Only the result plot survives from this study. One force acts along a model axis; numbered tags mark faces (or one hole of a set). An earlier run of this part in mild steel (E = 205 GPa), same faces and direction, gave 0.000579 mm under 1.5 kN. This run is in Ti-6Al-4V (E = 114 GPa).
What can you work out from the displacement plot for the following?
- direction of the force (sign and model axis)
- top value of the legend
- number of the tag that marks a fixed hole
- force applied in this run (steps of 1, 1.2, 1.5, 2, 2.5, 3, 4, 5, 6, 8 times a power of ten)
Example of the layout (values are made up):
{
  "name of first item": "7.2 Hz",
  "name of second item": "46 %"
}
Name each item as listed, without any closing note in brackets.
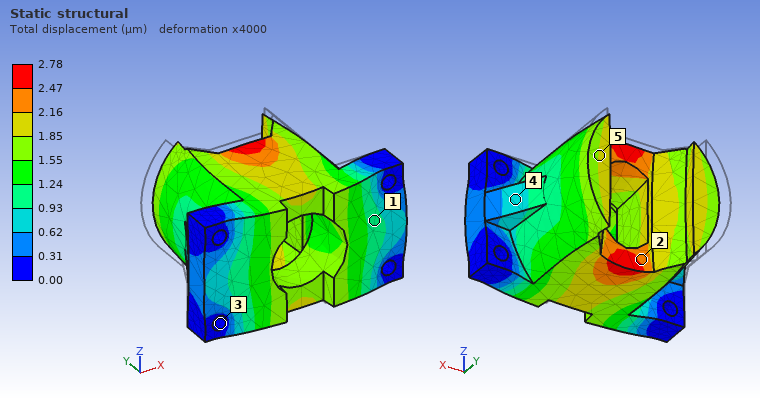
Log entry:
{
  "direction of the force": "-Y",
  "top value of the legend": "2.78 µm",
  "number of the tag that marks a fixed hole": "3",
  "force applied in this run": "4 kN"
}
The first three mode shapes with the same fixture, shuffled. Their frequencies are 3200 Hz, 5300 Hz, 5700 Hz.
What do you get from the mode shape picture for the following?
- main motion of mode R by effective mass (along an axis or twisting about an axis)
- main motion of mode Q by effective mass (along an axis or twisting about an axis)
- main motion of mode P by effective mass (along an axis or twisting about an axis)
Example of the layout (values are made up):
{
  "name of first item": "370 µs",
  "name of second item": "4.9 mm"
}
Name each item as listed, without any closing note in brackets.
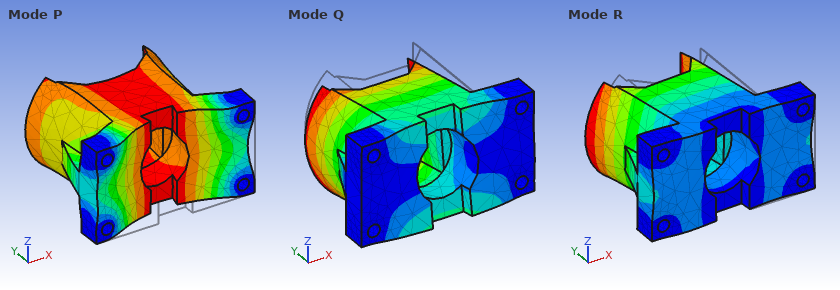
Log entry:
{
  "main motion of mode R by effective mass": "along X",
  "main motion of mode Q by effective mass": "along Z",
  "main motion of mode P by effective mass": "along Y"
}
